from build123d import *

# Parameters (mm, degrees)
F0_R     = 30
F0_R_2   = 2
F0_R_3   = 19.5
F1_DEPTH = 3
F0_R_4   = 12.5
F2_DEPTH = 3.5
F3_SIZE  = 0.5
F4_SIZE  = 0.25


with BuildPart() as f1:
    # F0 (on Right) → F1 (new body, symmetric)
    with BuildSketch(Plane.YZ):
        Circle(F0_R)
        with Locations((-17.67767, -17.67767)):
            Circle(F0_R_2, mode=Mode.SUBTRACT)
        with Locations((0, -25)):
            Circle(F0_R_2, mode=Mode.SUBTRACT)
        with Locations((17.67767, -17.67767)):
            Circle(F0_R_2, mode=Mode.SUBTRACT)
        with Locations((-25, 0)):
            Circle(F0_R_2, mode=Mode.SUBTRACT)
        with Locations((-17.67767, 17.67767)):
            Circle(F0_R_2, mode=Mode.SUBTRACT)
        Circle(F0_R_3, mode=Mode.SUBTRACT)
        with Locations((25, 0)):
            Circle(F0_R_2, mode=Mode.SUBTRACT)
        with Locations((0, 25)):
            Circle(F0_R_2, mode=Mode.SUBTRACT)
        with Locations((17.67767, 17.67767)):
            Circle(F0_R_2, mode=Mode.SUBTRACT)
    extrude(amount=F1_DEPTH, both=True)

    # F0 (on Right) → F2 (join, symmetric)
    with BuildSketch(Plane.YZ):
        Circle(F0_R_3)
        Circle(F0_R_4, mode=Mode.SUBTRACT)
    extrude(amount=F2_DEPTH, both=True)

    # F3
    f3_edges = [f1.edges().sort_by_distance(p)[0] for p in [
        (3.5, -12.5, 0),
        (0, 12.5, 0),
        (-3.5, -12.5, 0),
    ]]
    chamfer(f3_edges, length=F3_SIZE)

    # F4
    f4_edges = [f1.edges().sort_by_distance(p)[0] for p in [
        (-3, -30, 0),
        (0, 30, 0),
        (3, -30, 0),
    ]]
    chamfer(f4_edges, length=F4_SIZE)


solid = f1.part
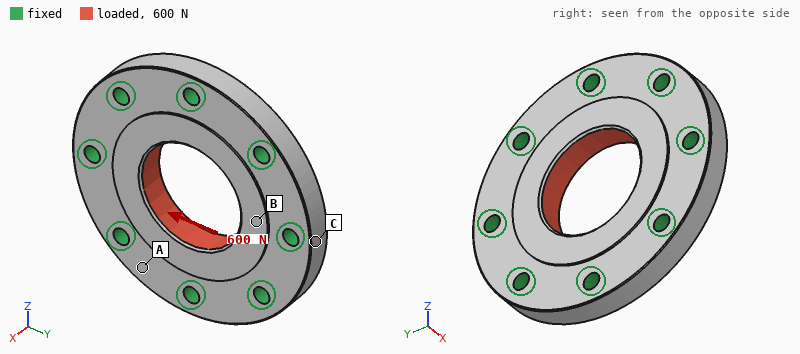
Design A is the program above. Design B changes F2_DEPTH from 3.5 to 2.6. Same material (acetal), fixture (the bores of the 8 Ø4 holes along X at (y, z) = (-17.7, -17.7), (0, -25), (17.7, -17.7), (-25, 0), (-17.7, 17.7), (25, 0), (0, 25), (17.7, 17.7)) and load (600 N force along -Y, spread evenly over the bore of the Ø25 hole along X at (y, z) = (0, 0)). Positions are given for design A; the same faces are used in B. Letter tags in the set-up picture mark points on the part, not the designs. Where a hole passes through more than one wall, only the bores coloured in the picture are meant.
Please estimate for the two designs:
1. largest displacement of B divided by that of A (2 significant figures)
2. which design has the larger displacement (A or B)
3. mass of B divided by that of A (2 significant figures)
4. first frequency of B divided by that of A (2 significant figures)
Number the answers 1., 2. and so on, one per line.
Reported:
1. 1.2
2. B
3. 0.91
4. 1.1
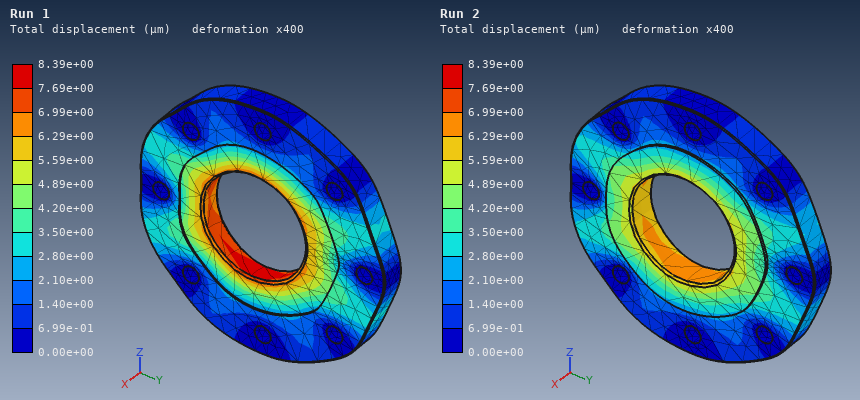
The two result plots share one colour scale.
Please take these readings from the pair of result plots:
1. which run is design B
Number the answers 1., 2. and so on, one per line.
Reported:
1. Run 1
